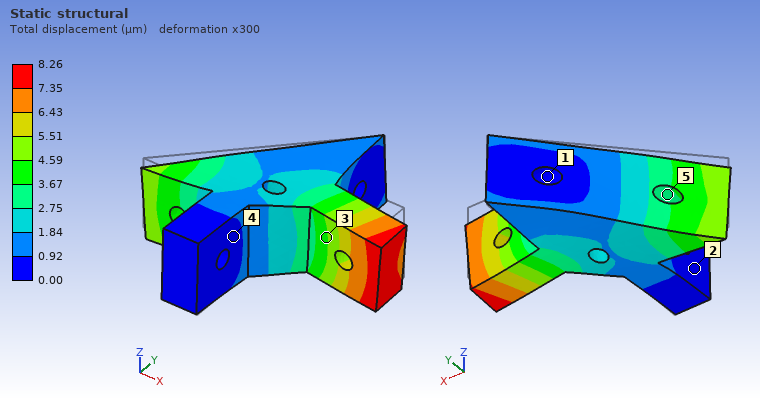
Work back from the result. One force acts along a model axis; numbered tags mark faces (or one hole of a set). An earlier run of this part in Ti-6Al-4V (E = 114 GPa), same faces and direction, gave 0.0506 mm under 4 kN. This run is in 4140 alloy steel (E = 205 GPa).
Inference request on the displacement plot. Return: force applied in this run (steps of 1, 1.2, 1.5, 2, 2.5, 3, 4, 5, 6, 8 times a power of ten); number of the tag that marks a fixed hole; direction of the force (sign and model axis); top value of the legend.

1.2 kN
1
-Z
8.26 µm
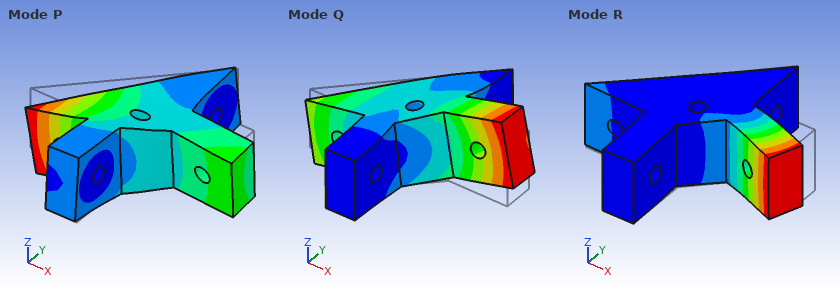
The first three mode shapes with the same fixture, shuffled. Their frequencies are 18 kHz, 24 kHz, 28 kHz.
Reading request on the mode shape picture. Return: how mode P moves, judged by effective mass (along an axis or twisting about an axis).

along Z
